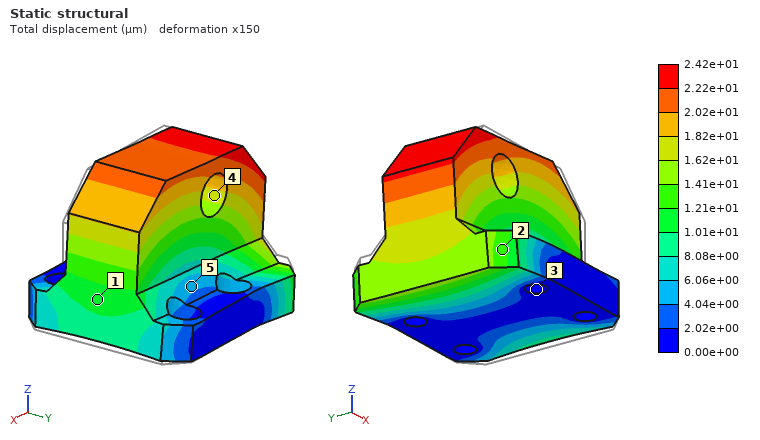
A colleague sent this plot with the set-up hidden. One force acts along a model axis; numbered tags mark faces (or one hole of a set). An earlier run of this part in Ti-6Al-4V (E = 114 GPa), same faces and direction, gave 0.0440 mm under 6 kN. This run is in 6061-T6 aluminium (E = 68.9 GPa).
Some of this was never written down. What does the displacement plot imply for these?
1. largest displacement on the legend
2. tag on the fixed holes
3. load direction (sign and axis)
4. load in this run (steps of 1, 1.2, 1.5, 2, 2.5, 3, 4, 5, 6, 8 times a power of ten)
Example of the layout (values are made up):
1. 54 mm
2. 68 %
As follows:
1. 2.42e+01 µm
2. 3
3. -X
4. 2 kN
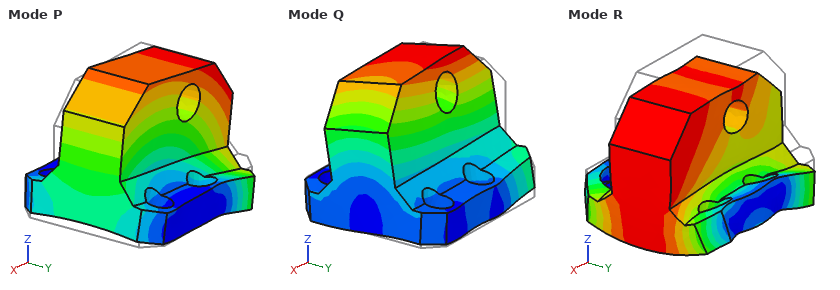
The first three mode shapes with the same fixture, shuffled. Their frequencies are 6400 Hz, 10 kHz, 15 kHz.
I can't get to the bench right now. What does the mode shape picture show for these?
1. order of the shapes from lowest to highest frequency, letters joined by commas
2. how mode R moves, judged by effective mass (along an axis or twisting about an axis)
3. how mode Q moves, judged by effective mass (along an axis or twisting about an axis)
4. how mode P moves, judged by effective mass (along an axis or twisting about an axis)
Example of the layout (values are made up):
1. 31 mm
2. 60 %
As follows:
1. P, Q, R
2. along Z
3. along Y
4. along X
